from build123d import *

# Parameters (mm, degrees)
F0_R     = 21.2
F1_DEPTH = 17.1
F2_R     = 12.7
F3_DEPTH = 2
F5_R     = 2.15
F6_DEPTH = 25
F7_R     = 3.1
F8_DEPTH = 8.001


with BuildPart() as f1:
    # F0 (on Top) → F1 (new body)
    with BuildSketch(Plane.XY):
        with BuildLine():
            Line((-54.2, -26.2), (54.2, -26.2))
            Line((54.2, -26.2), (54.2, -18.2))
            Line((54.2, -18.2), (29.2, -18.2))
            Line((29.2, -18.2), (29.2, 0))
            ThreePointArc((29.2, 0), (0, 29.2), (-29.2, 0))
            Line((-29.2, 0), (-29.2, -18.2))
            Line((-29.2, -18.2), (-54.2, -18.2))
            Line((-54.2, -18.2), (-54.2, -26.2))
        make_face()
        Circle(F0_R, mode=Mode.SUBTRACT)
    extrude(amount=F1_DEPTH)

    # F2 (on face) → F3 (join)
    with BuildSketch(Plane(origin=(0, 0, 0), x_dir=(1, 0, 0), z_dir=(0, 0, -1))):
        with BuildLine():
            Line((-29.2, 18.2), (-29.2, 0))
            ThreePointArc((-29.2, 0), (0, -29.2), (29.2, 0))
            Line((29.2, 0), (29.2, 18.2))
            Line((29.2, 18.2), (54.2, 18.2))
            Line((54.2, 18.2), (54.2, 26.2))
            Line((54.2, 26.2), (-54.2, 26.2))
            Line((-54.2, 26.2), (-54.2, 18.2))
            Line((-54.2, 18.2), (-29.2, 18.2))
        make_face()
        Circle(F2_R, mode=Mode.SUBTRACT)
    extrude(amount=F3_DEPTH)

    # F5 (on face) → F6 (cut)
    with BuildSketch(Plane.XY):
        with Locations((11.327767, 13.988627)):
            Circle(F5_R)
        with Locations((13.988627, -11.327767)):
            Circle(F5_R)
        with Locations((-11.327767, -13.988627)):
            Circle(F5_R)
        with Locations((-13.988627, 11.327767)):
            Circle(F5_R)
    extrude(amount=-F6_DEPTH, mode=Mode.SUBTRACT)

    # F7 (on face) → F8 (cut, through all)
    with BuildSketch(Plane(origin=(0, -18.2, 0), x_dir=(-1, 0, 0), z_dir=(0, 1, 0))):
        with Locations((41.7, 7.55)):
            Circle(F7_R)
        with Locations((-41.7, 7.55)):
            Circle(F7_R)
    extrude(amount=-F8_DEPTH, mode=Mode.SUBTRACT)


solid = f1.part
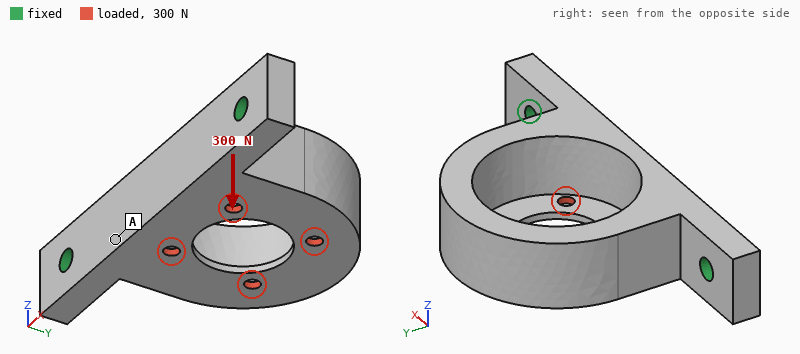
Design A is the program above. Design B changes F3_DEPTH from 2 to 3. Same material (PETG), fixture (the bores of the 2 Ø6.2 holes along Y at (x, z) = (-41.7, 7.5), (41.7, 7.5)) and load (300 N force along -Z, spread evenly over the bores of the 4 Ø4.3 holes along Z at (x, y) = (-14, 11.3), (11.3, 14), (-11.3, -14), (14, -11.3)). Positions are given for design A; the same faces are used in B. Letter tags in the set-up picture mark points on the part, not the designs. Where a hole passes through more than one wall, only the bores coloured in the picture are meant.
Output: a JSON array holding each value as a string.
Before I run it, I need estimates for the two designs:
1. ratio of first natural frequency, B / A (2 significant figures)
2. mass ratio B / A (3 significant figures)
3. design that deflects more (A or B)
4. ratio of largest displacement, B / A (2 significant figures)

["1.0", "1.07", "A", "0.91"]
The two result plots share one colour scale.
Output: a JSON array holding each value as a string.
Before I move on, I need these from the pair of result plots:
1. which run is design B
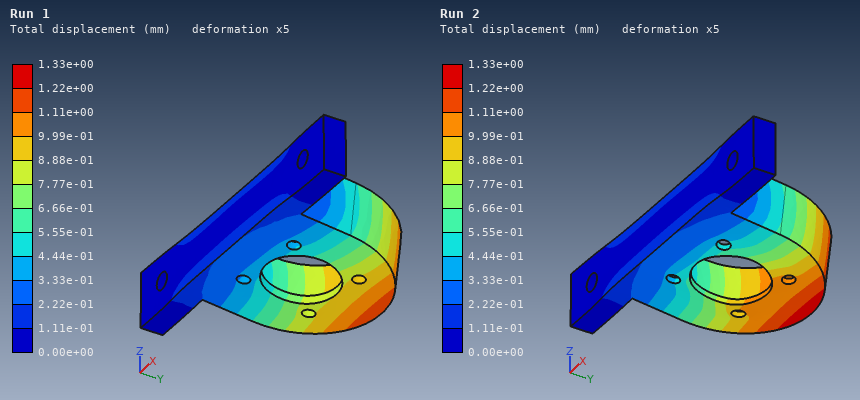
["Run 1"]
